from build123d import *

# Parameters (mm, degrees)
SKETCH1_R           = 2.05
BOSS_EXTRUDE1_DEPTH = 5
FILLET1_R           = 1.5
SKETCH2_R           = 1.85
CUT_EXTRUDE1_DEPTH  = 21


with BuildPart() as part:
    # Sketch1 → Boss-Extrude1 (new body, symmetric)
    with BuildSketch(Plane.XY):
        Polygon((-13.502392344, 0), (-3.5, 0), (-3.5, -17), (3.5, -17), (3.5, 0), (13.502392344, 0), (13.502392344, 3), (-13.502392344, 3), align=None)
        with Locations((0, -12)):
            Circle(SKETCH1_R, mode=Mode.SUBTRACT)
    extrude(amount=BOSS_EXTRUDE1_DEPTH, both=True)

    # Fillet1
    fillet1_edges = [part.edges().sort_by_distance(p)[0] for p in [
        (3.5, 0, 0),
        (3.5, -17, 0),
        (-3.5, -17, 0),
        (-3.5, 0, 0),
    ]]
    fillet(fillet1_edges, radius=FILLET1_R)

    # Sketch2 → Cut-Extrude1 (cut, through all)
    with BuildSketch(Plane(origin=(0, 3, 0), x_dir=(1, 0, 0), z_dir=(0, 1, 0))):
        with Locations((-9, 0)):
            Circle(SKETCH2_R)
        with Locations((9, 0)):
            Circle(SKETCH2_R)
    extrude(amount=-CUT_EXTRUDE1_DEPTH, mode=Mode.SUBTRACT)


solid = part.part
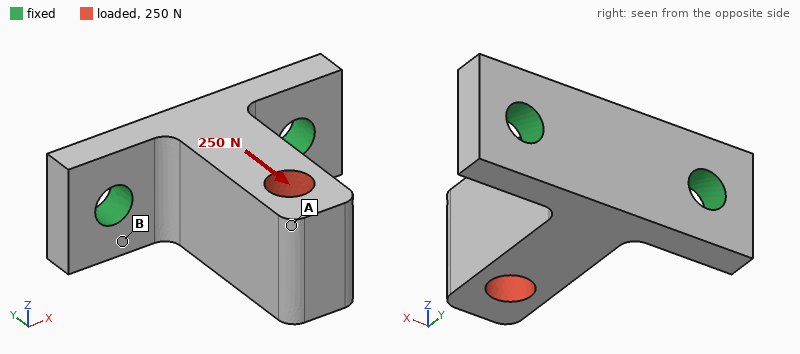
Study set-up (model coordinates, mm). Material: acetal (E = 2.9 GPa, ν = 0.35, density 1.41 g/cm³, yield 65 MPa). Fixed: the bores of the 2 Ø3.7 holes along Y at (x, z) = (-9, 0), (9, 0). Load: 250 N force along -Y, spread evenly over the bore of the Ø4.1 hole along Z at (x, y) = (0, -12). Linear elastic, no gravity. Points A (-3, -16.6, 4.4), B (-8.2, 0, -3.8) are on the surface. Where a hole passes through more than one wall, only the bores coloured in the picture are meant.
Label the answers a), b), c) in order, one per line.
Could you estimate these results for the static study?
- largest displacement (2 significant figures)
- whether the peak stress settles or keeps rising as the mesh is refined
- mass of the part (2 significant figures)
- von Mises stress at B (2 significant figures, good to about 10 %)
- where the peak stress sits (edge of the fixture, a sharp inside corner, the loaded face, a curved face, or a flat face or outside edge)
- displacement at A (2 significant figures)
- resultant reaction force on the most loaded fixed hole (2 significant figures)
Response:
a) 72 µm
b) keeps rising
c) 2.5 g
d) 6.0 MPa
e) edge of the fixture
f) 67 µm
g) 130 N
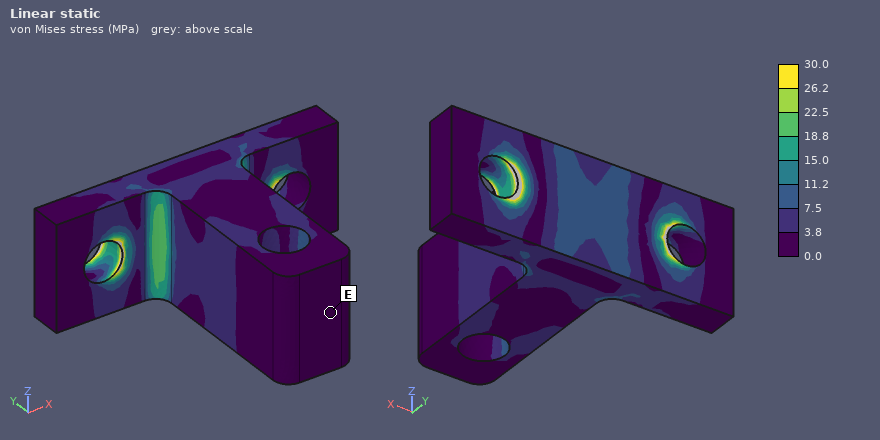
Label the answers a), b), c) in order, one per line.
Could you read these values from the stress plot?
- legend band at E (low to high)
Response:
a) 0.0 to 3.8 MPa
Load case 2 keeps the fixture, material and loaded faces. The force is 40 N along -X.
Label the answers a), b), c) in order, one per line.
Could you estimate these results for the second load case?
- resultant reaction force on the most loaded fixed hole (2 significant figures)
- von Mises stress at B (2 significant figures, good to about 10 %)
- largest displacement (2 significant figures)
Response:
a) 47 N
b) 1.1 MPa
c) 0.11 mm
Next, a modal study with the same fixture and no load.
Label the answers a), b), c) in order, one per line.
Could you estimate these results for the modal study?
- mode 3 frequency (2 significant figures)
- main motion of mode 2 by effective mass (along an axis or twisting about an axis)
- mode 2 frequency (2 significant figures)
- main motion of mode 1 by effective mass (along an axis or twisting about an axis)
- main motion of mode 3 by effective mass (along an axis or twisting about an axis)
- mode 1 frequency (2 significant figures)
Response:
a) 7900 Hz
b) along X
c) 3800 Hz
d) along Z
e) along Y
f) 2400 Hz
